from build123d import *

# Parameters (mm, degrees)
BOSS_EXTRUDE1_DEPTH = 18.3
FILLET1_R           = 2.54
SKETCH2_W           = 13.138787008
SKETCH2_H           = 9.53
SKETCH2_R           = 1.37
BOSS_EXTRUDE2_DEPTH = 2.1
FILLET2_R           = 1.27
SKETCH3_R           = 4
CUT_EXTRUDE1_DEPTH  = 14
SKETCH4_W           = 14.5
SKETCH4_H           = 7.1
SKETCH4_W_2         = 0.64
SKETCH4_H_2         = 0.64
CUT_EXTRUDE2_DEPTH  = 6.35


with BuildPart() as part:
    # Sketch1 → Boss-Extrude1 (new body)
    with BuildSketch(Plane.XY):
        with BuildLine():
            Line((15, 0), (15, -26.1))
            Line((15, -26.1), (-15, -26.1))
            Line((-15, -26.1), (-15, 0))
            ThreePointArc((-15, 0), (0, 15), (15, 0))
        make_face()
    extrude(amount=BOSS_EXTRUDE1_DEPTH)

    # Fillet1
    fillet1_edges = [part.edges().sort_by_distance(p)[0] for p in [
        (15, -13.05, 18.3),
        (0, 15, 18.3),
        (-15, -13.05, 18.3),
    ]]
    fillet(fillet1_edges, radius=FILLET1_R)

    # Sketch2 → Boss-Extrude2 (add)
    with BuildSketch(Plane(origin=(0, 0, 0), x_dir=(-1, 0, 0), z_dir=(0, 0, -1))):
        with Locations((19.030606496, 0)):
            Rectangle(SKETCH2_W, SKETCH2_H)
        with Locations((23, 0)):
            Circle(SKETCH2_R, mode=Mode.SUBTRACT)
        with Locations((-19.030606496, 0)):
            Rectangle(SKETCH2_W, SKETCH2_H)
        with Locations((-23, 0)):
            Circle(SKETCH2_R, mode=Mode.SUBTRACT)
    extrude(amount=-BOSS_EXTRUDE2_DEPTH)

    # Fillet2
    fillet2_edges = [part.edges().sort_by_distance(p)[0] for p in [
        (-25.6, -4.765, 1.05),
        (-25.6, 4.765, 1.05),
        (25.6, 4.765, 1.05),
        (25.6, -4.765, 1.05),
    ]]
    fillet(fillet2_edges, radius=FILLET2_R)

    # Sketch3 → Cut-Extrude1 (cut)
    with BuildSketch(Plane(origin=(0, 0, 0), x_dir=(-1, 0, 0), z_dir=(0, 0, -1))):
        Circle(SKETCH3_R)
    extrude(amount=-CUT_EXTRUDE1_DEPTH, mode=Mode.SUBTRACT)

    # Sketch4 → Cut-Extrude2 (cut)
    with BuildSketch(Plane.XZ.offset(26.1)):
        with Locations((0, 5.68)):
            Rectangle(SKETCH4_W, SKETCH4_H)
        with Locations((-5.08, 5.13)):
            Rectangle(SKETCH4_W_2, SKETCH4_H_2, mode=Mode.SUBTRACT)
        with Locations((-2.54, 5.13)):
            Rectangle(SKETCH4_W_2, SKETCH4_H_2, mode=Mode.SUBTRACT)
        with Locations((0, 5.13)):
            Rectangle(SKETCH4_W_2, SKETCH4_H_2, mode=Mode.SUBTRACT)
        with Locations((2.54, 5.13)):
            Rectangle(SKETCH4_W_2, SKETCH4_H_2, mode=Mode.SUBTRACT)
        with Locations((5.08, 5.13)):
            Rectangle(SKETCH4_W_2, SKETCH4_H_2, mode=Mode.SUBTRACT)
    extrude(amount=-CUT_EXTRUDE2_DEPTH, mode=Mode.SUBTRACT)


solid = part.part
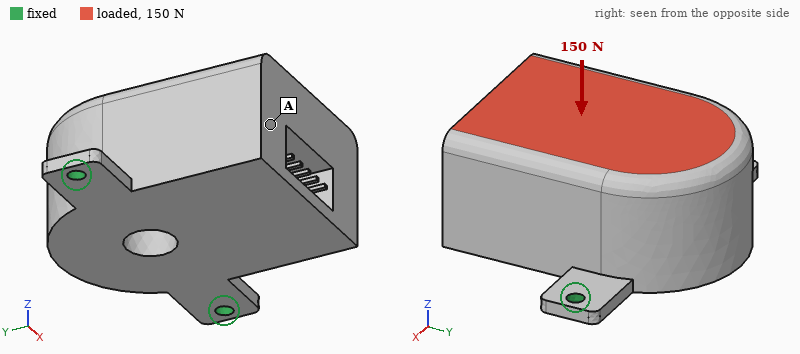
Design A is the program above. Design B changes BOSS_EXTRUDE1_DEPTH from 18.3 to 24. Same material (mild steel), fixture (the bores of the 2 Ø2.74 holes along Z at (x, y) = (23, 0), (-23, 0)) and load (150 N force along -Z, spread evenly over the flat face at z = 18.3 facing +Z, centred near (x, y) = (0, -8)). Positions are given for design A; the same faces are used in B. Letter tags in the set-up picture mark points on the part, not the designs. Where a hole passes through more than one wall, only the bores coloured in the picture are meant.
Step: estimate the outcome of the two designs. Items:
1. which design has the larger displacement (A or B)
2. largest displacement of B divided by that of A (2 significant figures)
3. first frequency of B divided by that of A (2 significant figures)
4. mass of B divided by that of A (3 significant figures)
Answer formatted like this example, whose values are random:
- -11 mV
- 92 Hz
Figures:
- B
- 1.1
- 0.76
- 1.33
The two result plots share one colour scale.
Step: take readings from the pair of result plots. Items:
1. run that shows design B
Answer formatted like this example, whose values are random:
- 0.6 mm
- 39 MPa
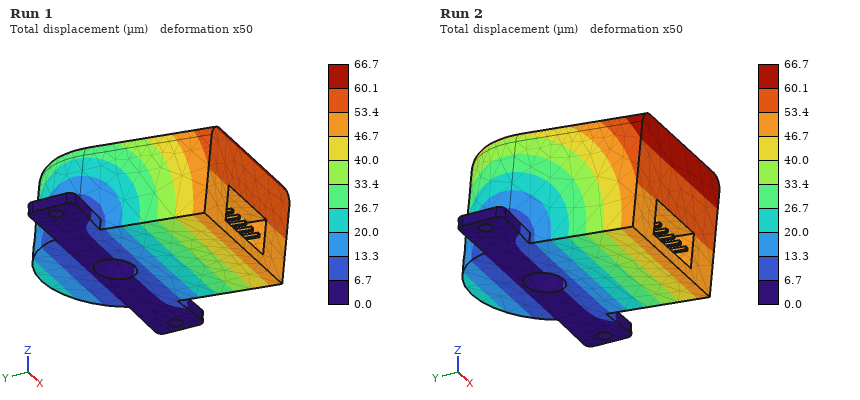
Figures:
- Run 2
